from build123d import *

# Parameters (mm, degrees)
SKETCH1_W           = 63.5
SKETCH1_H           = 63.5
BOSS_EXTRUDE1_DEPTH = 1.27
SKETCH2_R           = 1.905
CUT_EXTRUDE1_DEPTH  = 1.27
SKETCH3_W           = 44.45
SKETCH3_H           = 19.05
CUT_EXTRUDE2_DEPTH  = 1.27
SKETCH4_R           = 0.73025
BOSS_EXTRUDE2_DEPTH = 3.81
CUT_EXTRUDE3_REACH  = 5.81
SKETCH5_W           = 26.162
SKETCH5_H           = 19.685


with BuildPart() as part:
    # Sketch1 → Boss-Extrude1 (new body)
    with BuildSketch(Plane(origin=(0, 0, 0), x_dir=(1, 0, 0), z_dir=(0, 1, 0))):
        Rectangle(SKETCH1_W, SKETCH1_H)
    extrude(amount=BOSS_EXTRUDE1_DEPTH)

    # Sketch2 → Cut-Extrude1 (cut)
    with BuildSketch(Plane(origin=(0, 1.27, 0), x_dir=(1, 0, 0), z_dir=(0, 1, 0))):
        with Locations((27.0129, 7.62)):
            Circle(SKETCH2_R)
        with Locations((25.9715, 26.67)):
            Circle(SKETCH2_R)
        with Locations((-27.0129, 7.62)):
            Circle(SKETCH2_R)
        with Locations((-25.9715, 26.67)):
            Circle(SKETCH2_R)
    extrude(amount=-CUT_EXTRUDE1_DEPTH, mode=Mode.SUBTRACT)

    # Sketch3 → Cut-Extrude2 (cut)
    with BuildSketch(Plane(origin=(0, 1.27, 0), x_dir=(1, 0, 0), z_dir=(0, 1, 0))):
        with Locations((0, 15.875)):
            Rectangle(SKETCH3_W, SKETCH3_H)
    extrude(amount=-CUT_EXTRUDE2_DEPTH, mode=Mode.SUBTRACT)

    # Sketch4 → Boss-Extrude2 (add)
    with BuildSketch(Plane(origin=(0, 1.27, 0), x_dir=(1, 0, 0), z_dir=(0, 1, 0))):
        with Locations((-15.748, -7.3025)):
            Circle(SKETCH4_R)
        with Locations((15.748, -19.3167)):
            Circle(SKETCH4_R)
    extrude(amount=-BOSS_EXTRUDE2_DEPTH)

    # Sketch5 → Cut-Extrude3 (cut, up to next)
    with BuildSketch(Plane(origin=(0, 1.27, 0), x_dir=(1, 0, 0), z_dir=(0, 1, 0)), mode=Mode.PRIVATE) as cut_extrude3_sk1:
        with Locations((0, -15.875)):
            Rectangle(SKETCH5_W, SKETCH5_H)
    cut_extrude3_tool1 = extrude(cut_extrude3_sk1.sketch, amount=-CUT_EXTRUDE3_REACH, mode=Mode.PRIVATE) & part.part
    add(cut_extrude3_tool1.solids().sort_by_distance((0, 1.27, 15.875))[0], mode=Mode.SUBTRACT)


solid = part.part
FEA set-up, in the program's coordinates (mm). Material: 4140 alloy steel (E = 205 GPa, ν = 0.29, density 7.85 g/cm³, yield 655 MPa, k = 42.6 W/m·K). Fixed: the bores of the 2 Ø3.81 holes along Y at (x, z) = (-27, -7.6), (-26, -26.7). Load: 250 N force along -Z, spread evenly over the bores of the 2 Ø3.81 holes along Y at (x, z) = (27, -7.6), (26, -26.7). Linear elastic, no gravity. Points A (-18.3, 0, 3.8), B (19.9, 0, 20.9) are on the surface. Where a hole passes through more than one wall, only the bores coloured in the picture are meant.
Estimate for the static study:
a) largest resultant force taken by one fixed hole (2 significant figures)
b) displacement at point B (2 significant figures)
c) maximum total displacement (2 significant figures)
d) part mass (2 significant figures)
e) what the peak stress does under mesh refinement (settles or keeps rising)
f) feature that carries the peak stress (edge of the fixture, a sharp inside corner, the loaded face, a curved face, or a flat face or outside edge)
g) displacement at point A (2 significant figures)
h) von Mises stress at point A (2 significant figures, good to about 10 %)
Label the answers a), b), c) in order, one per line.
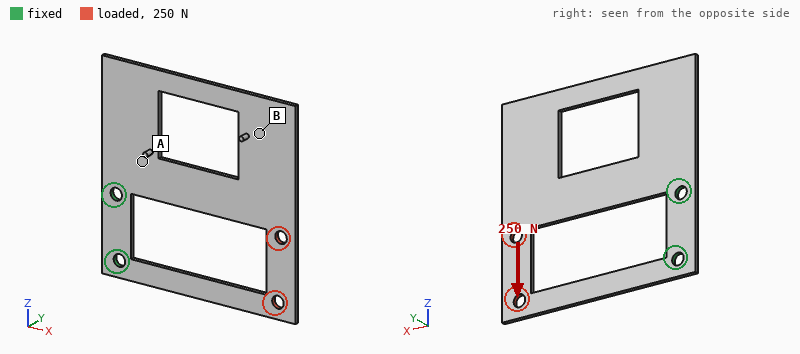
a) 400 N
b) 0.17 mm
c) 0.21 mm
d) 26 g
e) keeps rising
f) a sharp inside corner
g) 0.036 mm
h) 54 MPa
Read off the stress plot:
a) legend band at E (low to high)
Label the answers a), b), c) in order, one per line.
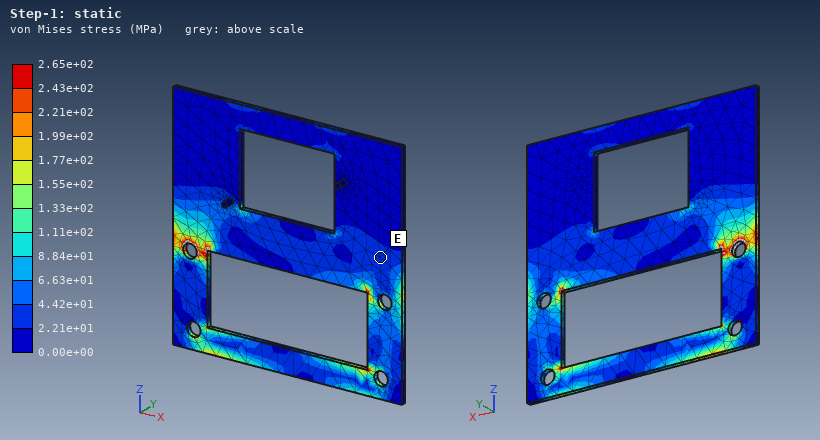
a) 2.21e+01 to 4.42e+01 MPa
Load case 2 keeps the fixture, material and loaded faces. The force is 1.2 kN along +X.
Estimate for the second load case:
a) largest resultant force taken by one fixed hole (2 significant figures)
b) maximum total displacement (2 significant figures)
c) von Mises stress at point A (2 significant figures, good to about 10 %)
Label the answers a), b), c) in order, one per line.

a) 610 N
b) 26 µm
c) 17 MPa
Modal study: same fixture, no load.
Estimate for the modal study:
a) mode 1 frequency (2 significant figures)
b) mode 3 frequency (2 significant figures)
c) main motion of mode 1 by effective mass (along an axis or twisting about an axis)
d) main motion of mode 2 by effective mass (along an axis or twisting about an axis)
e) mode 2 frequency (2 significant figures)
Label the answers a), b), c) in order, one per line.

a) 190 Hz
b) 860 Hz
c) along Y
d) twisting about X
e) 420 Hz
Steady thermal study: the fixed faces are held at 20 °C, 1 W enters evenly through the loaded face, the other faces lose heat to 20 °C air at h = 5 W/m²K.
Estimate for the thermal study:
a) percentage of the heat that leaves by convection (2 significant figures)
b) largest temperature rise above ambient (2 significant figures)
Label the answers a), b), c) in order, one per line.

a) 42 %
b) 39 K
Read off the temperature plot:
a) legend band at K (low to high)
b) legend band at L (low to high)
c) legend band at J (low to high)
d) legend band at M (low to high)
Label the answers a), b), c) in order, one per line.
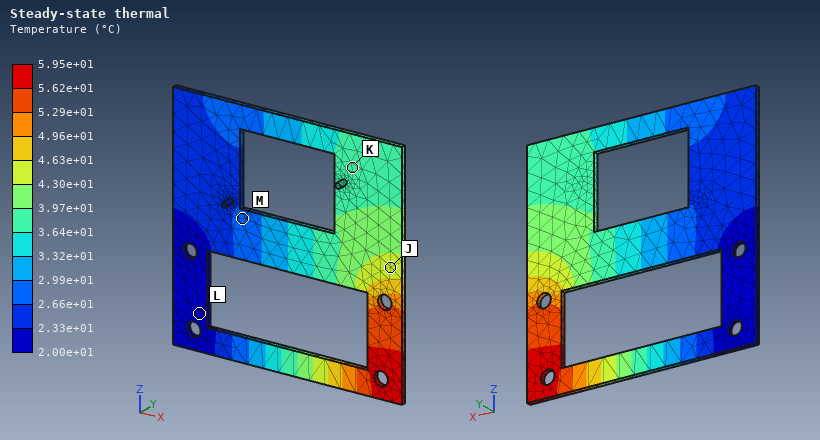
a) 3.64e+01 to 3.97e+01 °C
b) 2.00e+01 to 2.33e+01 °C
c) 4.30e+01 to 4.63e+01 °C
d) 2.66e+01 to 2.99e+01 °C
